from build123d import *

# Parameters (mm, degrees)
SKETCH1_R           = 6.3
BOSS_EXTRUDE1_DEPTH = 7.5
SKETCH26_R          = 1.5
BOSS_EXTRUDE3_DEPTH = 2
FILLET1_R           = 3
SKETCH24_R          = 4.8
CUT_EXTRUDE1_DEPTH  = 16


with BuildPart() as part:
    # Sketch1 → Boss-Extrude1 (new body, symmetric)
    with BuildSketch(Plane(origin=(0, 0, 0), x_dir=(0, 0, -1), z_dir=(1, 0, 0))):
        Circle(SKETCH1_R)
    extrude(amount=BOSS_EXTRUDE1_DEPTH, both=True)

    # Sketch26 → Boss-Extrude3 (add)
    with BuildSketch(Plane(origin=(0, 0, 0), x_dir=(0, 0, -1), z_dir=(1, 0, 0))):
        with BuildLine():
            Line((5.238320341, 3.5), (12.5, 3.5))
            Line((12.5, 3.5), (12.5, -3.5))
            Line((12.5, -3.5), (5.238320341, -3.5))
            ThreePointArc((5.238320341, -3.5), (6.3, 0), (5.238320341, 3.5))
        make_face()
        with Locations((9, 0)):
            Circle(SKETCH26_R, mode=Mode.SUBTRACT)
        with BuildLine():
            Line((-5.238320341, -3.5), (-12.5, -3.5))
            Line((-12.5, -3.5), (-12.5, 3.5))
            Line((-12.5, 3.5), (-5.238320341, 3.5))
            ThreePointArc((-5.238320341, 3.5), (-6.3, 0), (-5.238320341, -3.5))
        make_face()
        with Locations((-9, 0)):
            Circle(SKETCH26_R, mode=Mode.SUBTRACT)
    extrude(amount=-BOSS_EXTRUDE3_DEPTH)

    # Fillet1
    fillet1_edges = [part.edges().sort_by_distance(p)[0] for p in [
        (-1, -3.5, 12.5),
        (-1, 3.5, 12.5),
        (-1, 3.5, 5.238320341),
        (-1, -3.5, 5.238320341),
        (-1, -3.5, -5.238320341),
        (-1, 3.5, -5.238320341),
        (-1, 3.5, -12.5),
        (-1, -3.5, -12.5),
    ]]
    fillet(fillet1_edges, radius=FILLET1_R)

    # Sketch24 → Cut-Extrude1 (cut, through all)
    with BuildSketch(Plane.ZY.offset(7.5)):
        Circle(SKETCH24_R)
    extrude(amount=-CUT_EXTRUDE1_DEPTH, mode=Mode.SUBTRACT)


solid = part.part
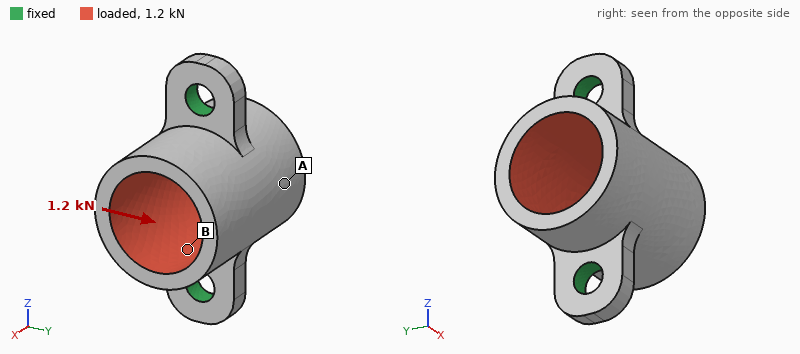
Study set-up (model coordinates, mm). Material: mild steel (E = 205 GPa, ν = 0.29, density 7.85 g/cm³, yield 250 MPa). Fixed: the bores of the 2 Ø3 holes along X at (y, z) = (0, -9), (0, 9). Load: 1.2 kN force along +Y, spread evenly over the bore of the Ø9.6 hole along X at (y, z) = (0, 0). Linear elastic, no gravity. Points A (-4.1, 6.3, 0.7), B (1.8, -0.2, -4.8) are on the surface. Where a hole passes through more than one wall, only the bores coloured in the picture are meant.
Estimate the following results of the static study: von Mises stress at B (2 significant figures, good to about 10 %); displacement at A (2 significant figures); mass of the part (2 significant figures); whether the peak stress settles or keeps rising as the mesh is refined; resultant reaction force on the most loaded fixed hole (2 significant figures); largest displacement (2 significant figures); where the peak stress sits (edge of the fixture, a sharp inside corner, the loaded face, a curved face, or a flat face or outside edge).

38 MPa
5.3 µm
7.3 g
keeps rising
600 N
13 µm
edge of the fixture
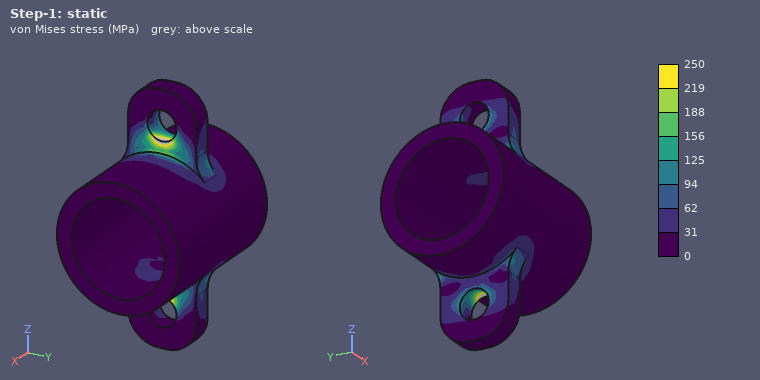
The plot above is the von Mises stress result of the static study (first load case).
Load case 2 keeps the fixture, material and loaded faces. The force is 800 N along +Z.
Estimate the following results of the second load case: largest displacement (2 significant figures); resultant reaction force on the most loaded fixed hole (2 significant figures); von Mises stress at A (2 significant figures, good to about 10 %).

2.3 µm
400 N
11 MPa
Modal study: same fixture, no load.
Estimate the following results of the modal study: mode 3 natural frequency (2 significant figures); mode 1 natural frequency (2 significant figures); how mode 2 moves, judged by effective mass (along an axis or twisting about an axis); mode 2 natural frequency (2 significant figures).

39 kHz
13 kHz
along X
28 kHz
